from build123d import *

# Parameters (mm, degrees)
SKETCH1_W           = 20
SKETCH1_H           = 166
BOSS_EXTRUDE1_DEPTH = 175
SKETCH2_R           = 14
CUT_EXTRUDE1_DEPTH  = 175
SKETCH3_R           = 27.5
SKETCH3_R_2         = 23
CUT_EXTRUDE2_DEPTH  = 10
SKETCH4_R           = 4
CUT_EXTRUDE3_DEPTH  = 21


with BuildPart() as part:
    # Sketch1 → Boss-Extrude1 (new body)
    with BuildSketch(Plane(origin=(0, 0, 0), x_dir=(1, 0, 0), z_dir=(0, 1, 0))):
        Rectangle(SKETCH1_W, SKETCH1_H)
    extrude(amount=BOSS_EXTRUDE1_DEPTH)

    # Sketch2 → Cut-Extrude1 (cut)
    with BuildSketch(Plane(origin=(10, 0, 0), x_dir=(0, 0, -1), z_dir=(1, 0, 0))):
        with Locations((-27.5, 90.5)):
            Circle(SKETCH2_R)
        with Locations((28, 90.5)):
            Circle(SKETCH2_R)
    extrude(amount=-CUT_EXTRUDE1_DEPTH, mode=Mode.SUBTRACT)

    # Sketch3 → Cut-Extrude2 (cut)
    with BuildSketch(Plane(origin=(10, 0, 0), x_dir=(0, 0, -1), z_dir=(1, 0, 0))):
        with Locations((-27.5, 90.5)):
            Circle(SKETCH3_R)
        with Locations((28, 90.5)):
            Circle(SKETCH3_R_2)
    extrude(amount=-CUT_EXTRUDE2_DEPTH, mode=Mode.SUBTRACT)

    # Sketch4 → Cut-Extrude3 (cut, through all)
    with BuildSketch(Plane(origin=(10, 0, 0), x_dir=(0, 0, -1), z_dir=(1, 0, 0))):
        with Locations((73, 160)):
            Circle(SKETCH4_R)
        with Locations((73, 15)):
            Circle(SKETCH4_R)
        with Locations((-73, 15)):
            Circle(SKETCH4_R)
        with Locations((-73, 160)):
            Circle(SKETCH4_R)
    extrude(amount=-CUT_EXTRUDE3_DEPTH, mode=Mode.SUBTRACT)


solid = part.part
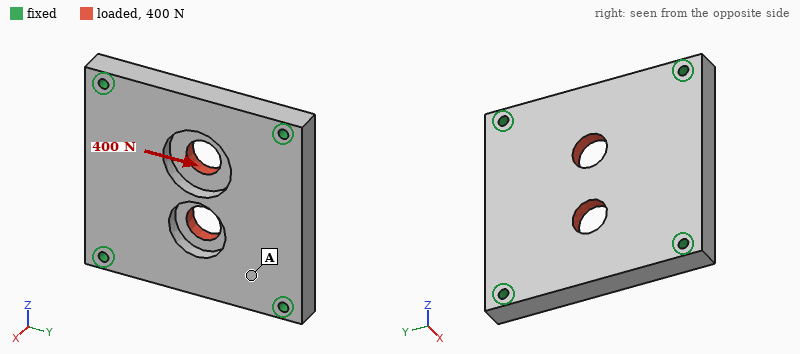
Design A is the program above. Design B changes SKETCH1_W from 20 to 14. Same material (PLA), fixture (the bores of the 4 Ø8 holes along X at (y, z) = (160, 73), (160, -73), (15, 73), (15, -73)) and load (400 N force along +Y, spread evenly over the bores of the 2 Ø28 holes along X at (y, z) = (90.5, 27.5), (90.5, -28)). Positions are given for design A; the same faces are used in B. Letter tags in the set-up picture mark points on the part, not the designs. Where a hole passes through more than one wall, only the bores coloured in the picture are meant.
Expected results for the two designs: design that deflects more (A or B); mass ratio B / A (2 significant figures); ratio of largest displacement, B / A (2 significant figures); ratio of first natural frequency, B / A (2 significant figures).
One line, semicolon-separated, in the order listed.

B; 0.70; 1.4; 0.75
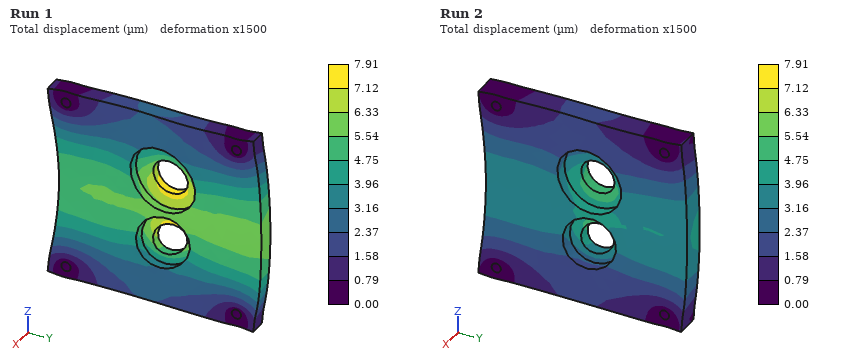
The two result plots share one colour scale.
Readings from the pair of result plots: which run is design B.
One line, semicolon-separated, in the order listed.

Run 1
